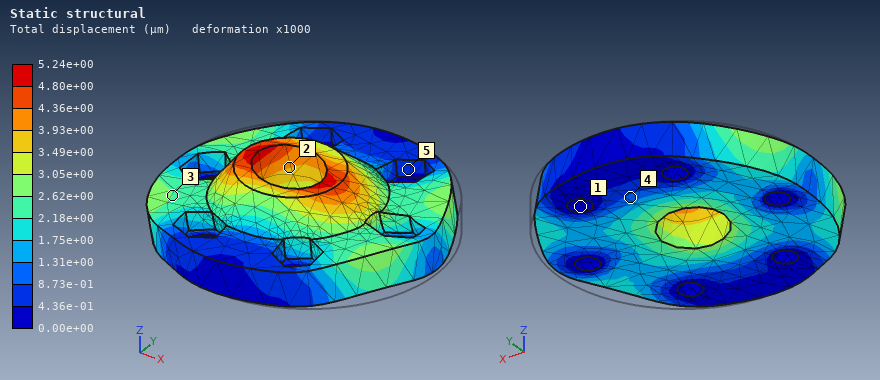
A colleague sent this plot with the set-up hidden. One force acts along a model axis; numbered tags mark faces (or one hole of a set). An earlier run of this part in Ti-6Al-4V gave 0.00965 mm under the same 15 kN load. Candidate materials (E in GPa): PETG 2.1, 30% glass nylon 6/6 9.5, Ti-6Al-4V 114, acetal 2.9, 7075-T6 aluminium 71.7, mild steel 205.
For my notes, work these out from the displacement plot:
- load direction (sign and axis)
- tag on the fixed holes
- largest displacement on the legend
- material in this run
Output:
-X
1
5.24e+00 µm
mild steel
